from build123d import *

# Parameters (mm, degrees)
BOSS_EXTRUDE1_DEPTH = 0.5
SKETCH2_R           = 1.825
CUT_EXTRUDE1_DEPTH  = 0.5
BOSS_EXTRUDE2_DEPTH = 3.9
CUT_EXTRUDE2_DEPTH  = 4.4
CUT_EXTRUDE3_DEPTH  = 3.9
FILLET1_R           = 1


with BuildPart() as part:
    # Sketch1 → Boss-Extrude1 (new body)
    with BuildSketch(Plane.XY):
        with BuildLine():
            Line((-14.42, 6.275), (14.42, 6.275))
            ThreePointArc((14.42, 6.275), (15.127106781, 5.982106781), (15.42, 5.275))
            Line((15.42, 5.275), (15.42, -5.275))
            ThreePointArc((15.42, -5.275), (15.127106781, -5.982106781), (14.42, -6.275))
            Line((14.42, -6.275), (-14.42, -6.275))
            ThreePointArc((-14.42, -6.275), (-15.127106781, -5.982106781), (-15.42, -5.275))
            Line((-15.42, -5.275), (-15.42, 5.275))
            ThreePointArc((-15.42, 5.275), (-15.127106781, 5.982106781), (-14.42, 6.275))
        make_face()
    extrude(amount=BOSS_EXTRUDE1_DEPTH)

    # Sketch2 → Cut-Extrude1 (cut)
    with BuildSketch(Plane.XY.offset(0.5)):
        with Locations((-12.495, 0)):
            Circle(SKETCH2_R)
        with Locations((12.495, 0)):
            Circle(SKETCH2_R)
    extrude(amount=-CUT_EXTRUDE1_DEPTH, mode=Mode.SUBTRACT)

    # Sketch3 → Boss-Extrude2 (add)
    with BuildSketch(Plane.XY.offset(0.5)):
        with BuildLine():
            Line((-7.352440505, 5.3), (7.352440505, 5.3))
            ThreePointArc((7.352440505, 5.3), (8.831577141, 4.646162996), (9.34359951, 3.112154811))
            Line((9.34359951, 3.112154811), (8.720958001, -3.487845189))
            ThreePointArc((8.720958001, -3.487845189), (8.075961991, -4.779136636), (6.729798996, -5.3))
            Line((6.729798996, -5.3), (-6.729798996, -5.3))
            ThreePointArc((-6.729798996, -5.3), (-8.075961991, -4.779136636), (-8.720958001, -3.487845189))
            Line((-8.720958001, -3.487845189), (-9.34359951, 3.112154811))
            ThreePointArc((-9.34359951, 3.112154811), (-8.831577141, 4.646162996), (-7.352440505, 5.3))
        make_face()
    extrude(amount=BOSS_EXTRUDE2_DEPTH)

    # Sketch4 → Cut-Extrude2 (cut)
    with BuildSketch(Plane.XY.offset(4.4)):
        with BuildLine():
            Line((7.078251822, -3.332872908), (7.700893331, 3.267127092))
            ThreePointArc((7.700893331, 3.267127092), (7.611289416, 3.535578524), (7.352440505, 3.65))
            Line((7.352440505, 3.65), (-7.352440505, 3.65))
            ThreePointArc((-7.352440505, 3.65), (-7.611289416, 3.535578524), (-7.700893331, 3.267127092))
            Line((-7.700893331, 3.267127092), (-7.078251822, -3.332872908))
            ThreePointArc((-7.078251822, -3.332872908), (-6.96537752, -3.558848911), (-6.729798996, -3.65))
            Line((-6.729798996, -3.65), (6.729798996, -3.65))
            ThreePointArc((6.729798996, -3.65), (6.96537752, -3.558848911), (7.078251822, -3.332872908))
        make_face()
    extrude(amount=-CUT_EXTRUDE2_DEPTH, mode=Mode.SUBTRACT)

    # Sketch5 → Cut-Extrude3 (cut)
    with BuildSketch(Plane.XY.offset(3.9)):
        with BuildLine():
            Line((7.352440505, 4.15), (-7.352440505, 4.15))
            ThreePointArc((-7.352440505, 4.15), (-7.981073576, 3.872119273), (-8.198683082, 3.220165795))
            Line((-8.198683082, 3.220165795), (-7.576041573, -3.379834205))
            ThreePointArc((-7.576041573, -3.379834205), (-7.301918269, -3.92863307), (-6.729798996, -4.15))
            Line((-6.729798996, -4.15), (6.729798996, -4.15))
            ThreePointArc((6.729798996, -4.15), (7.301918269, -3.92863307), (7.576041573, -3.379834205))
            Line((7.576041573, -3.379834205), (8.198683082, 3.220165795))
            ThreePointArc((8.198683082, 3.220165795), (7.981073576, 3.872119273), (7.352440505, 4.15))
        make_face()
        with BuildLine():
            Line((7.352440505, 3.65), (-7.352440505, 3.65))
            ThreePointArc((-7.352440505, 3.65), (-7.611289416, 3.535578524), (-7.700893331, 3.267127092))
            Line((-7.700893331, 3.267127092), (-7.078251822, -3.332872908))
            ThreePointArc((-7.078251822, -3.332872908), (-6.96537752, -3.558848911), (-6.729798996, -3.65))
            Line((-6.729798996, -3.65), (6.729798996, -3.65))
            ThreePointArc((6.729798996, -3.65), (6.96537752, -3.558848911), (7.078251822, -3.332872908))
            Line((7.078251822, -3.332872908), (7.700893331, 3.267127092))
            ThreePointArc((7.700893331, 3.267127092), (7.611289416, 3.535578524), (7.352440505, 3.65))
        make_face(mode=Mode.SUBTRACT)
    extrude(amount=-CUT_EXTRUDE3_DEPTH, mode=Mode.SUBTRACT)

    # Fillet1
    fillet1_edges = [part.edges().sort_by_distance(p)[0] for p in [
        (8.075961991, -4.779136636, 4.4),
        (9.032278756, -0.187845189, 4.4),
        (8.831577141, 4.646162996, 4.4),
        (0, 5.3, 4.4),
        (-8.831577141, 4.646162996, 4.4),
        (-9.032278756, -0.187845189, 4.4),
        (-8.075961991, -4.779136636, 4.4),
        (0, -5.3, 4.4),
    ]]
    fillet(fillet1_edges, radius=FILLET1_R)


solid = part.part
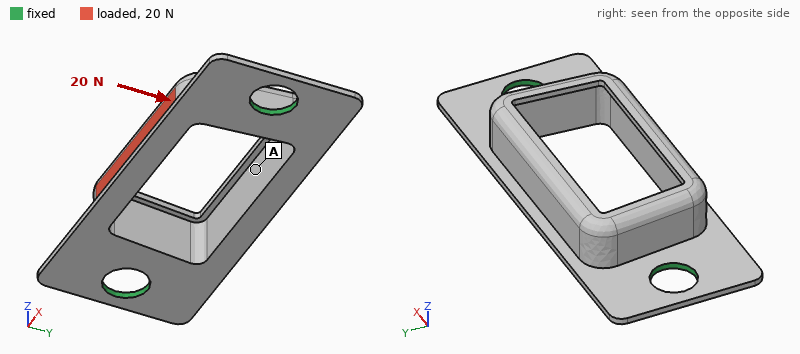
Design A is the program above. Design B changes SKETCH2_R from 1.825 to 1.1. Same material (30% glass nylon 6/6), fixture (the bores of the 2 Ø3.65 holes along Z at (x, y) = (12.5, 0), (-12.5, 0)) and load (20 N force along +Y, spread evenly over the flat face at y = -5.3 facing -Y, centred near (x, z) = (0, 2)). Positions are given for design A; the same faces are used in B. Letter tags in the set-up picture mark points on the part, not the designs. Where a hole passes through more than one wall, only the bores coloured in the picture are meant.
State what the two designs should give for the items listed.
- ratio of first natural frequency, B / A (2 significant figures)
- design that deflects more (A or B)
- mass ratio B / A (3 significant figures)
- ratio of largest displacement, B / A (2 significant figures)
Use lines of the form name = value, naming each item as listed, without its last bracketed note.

ratio of first natural frequency, B / A = 0.70
design that deflects more = B
mass ratio B / A = 1.02
ratio of largest displacement, B / A = 1.6
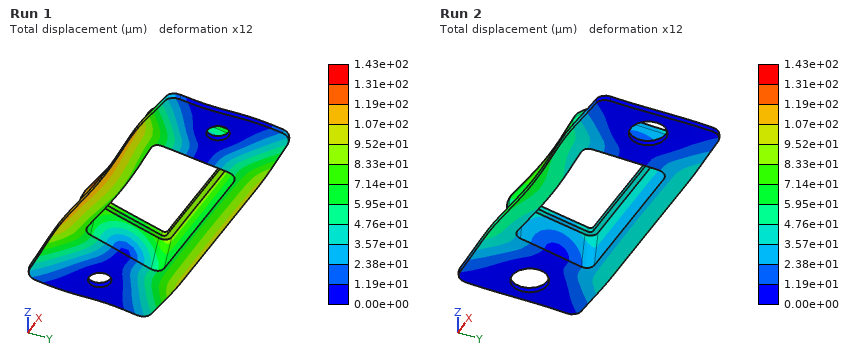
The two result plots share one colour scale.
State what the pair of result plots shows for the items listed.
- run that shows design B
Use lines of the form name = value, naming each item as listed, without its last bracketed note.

run that shows design B = Run 1
